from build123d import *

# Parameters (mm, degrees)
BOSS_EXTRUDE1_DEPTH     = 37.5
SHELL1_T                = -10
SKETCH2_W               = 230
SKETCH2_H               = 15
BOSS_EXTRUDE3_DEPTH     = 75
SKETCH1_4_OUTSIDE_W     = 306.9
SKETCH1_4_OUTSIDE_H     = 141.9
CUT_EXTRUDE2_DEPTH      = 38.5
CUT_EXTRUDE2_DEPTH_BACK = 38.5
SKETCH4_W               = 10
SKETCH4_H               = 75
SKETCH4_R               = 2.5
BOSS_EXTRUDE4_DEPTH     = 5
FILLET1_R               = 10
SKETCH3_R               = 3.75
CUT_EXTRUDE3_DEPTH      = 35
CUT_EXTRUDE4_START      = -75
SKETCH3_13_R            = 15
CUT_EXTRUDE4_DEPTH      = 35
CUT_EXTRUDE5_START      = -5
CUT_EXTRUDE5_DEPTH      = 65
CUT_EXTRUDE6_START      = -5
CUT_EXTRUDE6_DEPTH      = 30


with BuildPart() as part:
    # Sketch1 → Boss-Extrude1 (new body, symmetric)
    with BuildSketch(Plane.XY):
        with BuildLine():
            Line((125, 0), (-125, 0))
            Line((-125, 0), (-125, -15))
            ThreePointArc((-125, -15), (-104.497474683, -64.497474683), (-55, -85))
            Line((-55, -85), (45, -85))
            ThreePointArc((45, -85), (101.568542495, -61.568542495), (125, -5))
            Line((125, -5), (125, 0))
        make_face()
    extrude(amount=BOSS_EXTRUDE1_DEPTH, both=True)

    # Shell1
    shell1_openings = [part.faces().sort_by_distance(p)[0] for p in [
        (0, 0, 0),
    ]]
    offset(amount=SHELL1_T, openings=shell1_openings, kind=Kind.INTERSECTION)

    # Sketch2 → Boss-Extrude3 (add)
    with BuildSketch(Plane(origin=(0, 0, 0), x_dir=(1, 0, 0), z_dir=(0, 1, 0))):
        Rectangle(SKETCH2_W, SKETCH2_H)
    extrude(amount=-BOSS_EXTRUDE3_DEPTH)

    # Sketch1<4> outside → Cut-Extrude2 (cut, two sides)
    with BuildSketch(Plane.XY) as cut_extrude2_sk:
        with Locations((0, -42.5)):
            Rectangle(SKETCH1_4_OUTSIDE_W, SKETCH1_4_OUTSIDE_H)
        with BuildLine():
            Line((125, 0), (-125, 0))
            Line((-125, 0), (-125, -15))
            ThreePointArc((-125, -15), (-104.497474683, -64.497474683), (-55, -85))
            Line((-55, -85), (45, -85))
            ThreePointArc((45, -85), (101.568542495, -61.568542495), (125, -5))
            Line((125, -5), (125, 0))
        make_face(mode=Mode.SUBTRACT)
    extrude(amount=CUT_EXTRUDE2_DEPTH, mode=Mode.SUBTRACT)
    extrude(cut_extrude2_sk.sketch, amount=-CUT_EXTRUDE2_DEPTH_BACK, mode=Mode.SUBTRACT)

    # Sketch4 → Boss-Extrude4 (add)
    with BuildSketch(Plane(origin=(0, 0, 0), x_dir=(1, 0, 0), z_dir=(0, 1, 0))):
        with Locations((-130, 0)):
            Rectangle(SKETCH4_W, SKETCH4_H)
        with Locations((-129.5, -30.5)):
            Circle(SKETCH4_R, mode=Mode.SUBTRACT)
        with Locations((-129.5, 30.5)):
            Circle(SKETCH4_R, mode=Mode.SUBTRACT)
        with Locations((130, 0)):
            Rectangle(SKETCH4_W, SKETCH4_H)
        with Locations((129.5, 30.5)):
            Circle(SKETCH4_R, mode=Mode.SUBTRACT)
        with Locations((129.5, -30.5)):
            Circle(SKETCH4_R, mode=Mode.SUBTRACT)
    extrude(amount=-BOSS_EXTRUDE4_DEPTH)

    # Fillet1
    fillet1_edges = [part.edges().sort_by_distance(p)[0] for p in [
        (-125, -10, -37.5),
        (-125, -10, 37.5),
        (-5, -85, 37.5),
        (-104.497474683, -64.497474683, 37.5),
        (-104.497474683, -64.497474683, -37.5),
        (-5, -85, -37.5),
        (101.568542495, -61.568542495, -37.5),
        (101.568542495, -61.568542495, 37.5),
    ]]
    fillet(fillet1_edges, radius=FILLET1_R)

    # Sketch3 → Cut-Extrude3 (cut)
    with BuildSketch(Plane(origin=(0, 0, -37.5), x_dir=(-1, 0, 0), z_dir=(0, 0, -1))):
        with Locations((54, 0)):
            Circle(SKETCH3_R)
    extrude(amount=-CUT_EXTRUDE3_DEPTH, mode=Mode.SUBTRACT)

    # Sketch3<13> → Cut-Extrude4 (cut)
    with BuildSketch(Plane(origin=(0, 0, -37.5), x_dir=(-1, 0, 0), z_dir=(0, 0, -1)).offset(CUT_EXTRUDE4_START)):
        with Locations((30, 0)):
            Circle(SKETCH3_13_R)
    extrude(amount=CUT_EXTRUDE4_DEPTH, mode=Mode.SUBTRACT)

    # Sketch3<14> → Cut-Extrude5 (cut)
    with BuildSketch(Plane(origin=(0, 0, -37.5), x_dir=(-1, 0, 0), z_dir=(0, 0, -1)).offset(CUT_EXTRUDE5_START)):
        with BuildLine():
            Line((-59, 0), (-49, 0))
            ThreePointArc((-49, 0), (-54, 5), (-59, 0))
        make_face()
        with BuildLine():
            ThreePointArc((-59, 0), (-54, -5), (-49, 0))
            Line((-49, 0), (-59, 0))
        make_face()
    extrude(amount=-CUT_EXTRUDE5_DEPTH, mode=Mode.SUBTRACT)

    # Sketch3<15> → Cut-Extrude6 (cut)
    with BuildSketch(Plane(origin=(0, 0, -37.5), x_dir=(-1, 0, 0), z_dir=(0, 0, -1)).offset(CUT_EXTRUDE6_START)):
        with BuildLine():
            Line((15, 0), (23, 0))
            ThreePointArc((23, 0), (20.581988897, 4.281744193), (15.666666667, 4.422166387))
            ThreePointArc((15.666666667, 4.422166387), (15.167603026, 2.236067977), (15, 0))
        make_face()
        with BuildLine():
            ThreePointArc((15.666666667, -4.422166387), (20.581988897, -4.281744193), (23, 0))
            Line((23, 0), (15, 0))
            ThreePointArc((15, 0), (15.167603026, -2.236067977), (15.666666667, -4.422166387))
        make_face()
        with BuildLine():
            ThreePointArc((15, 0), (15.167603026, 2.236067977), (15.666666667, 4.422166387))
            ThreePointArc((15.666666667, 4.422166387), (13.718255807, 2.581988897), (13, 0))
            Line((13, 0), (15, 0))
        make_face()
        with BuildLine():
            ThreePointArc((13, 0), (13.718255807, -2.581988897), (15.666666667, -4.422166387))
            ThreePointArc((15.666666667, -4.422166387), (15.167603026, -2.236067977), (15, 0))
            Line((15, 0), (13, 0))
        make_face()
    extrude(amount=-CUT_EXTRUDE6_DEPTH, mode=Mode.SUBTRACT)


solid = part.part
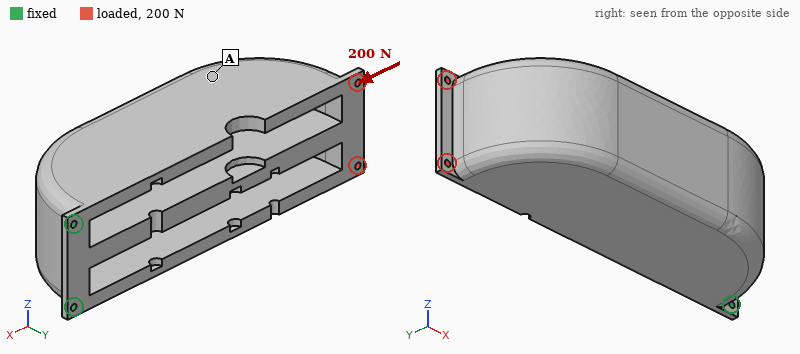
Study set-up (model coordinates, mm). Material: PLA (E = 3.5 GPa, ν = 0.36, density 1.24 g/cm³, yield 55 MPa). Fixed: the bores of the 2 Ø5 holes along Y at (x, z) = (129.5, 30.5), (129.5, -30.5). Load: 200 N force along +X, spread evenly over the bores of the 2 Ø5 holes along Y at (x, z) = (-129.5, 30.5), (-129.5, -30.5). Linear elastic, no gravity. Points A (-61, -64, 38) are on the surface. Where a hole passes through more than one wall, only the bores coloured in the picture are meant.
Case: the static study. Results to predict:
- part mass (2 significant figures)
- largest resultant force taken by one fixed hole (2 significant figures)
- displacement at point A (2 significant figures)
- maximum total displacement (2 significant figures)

970 g
100 N
0.096 mm
0.16 mm
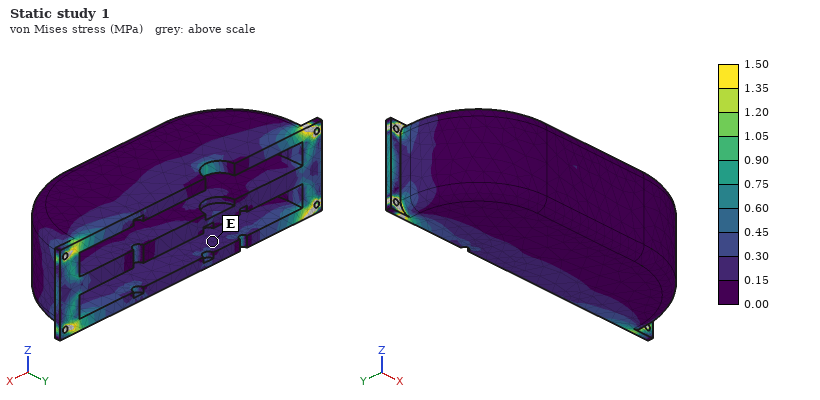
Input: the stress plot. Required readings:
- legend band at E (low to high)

0.15 to 0.30 MPa
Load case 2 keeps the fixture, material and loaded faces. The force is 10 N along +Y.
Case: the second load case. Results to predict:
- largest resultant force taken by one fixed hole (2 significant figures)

8.6 N
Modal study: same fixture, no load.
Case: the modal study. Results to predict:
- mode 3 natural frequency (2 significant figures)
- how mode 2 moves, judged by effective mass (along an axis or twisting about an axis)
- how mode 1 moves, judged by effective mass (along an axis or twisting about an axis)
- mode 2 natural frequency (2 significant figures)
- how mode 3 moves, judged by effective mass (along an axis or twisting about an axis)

320 Hz
along Z
along Y
83 Hz
along Z
